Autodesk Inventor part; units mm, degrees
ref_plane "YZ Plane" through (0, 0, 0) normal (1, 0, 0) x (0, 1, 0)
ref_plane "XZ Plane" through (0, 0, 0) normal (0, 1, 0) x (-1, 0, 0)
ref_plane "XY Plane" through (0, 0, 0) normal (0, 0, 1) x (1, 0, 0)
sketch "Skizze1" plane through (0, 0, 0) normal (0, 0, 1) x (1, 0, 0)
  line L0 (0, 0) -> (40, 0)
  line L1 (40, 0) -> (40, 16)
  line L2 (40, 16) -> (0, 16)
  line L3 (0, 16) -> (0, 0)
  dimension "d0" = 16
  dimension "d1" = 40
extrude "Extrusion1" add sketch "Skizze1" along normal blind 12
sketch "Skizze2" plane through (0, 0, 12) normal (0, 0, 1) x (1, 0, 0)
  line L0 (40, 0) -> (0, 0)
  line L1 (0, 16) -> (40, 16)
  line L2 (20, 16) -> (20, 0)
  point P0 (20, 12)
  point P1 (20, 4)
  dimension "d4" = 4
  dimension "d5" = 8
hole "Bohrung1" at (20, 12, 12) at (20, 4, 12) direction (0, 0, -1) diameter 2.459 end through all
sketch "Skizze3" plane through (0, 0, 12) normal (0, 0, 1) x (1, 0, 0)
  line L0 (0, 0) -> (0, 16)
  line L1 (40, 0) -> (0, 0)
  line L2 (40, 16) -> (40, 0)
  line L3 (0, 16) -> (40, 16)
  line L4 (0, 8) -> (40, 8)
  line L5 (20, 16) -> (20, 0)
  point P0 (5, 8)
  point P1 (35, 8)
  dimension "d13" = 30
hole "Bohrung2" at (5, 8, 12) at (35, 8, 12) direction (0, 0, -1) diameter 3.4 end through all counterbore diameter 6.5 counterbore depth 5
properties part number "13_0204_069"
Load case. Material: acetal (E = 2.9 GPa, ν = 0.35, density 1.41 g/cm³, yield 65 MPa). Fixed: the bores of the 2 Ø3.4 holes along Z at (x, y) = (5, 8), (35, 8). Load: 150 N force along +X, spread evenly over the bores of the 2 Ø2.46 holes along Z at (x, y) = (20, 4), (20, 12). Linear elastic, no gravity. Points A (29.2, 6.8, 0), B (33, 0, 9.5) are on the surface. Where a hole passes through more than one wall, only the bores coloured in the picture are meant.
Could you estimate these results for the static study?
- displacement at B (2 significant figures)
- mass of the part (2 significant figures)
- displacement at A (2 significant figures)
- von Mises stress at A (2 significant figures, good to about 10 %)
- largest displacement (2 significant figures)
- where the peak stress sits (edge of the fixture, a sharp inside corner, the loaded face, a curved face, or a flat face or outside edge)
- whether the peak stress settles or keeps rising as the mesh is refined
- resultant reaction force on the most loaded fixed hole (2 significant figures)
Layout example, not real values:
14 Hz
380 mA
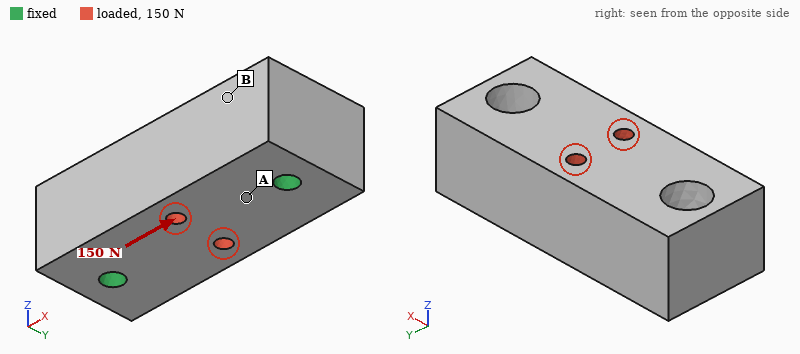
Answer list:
2.4 µm
10 g
1.5 µm
0.81 MPa
3.8 µm
edge of the fixture
keeps rising
76 N
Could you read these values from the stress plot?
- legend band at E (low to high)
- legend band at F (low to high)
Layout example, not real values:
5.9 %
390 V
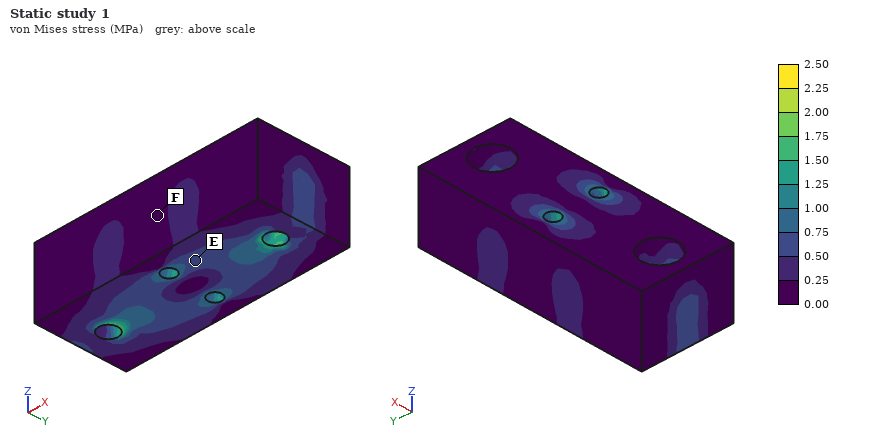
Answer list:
0.50 to 0.75 MPa
0.00 to 0.25 MPa
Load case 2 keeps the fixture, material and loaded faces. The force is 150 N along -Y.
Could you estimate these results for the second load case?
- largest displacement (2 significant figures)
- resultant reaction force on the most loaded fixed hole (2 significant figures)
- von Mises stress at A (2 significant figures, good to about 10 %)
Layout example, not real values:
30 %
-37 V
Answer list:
17 µm
75 N
0.90 MPa
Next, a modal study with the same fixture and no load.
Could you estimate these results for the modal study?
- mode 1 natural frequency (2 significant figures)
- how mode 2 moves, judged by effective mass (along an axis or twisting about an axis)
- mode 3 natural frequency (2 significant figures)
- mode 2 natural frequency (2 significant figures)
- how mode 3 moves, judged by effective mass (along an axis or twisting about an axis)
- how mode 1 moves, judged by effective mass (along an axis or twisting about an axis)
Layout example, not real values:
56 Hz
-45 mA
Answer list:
6700 Hz
along Z
9600 Hz
8300 Hz
along Y
along Y
